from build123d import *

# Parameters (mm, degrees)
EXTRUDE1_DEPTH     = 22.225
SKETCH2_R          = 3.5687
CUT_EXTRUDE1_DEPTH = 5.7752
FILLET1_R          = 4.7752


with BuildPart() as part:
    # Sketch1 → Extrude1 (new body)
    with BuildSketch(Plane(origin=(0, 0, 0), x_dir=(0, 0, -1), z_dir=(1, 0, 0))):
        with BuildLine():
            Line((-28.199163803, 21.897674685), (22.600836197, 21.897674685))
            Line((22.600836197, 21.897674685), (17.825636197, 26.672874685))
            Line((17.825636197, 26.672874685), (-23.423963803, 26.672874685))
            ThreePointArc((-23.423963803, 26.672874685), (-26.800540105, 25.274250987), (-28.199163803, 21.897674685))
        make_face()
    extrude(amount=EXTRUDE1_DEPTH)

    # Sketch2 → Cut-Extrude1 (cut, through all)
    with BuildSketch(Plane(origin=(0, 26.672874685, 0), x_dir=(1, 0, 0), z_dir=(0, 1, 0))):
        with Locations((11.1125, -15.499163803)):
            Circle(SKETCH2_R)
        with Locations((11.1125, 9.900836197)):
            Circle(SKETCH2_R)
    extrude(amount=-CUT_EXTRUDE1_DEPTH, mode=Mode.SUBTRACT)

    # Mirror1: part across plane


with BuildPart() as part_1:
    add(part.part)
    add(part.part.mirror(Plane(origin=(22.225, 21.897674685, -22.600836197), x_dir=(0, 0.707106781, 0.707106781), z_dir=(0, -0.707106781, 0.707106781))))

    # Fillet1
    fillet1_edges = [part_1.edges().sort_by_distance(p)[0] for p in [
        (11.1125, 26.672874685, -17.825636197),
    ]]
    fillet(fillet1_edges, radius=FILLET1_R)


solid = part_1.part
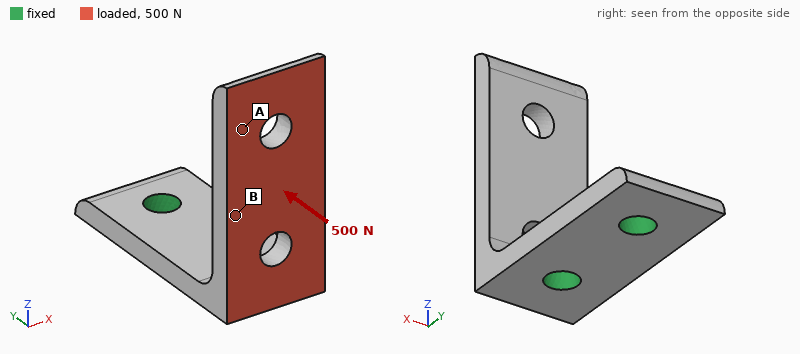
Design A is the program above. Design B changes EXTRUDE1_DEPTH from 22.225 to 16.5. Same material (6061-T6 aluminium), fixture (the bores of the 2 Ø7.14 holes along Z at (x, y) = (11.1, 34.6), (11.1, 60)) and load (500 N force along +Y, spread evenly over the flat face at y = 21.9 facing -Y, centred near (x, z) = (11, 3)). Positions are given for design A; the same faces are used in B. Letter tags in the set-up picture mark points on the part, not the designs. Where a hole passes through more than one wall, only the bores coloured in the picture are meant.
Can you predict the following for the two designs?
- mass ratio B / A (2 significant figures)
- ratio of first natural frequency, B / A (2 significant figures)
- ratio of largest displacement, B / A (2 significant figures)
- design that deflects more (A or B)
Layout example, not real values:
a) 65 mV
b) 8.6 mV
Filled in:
a) 0.72
b) 0.98
c) 1.4
d) B
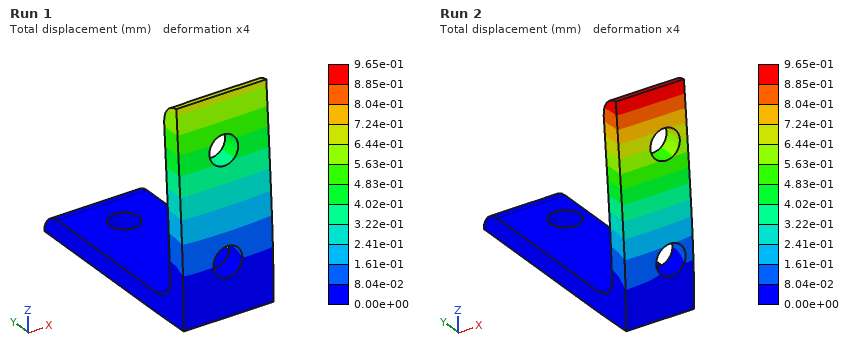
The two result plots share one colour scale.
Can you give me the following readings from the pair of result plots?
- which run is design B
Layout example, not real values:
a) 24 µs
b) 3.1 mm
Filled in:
a) Run 2
